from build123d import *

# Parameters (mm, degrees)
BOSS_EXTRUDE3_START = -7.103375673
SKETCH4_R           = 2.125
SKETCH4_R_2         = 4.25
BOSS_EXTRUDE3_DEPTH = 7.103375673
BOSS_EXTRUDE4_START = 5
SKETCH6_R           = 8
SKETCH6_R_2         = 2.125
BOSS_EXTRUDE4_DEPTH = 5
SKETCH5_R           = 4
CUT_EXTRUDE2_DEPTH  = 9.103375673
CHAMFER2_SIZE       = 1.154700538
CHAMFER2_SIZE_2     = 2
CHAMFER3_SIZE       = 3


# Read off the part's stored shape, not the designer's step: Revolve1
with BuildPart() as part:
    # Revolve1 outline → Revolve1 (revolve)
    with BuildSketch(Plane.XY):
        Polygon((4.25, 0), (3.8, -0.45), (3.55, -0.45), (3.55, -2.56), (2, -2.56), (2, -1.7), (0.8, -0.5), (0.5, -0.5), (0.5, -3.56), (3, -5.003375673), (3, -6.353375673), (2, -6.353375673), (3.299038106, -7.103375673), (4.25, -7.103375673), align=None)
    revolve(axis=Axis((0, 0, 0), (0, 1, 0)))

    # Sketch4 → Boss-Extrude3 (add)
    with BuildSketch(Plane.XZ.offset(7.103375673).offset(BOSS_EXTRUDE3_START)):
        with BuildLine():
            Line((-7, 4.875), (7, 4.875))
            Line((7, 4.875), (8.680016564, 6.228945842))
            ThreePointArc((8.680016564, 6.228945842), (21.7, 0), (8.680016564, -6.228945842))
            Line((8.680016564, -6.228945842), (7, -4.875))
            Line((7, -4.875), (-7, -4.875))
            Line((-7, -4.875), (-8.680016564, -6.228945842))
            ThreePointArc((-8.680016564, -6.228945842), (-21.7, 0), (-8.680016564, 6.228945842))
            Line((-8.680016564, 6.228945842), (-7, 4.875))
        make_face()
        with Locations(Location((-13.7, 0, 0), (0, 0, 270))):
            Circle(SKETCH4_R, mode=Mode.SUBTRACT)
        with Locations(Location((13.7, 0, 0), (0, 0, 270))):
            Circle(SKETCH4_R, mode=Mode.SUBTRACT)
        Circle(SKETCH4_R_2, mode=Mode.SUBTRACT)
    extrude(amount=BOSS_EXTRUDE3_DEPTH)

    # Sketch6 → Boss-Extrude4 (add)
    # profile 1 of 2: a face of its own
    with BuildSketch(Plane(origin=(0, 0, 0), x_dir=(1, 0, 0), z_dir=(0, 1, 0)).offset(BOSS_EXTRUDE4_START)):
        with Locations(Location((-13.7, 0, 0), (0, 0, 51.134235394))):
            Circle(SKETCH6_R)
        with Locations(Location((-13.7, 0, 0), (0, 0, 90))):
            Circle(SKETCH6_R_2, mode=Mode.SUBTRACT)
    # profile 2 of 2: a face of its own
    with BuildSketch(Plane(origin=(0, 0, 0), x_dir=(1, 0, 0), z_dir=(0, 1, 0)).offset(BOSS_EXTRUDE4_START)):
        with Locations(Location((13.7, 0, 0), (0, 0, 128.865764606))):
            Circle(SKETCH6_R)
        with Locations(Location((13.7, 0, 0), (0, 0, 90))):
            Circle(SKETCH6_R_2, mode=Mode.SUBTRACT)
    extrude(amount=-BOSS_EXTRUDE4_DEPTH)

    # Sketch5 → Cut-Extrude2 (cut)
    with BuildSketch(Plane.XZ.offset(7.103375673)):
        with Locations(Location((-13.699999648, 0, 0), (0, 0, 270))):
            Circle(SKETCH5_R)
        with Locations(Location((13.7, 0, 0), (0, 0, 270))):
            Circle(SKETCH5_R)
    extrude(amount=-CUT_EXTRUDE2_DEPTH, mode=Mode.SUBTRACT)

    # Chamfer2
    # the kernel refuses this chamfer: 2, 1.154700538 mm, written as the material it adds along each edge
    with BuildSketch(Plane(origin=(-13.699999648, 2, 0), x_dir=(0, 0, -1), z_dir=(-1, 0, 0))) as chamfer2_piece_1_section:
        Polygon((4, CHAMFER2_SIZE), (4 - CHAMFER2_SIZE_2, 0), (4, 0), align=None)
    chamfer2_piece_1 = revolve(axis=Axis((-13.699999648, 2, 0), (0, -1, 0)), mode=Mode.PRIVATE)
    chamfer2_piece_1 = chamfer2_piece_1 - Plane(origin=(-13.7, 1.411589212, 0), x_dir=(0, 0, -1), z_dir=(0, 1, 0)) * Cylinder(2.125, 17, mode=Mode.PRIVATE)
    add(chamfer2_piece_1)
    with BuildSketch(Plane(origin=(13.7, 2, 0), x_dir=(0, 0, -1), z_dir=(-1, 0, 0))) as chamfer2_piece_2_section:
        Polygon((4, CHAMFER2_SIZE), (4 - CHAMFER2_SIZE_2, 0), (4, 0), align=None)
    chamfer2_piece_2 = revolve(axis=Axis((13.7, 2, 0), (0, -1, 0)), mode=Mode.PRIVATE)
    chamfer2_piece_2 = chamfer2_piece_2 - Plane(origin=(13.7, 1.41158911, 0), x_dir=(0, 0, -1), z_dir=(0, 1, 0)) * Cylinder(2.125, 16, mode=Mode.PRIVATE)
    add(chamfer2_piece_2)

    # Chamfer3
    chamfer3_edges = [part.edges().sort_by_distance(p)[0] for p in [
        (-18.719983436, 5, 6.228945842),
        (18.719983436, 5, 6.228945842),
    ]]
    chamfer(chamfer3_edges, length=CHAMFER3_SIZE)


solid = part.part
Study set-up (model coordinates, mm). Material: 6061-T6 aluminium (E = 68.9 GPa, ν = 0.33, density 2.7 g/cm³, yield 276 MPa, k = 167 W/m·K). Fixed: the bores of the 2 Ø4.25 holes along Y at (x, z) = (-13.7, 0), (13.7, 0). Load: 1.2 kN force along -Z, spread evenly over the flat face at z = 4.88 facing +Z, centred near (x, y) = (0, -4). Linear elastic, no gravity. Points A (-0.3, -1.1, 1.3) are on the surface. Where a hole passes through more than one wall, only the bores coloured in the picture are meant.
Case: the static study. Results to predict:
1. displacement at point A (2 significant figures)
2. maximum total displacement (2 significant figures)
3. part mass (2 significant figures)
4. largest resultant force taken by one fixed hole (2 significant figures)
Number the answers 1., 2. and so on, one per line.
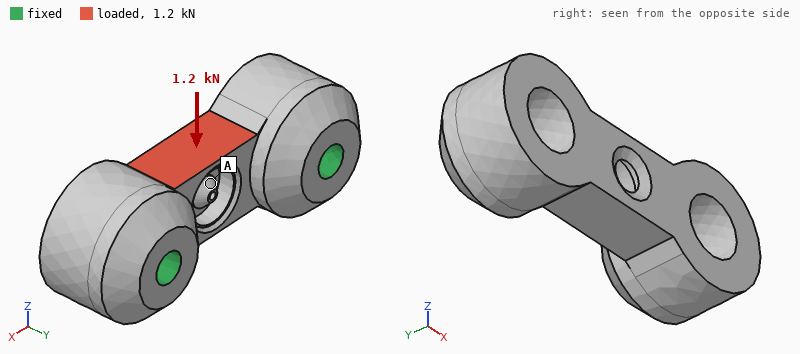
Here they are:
1. 15 µm
2. 27 µm
3. 11 g
4. 600 N
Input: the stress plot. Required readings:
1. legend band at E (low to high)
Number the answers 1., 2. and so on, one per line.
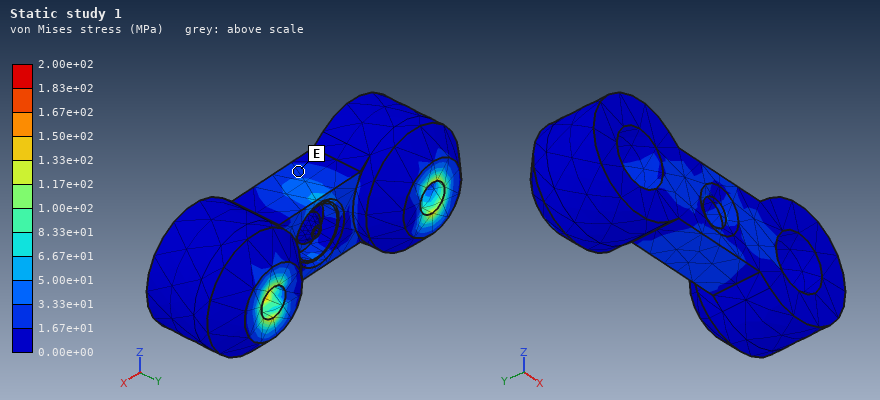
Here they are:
1. 1.67e+01 to 3.33e+01 MPa
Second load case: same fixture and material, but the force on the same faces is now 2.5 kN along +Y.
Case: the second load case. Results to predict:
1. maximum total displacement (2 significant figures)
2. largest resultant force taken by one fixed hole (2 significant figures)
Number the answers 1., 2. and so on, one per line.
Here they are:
1. 53 µm
2. 1.7 kN
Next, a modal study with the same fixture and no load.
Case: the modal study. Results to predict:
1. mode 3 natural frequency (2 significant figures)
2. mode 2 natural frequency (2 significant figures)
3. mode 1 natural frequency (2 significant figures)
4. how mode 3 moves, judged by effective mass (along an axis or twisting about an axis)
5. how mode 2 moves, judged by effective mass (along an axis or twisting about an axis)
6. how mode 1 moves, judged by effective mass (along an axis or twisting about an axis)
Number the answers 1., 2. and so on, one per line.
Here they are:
1. 27 kHz
2. 22 kHz
3. 16 kHz
4. along X
5. twisting about Y
6. along Z
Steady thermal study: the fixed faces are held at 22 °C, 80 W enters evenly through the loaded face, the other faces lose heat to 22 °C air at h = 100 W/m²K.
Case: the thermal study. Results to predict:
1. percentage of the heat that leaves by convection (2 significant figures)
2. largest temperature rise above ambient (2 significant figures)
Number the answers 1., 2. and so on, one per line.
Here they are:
1. 5.4 %
2. 63 K
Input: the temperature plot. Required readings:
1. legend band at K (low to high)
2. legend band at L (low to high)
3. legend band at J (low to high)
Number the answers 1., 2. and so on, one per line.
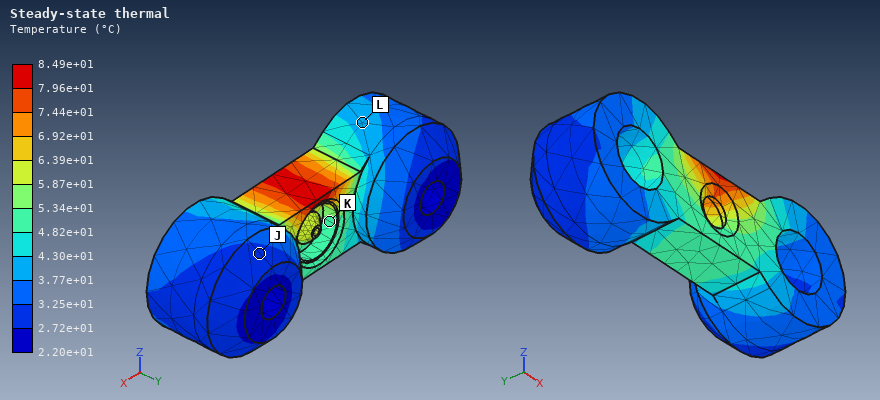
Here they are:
1. 4.82e+01 to 5.34e+01 °C
2. 3.77e+01 to 4.30e+01 °C
3. 2.72e+01 to 3.25e+01 °C
